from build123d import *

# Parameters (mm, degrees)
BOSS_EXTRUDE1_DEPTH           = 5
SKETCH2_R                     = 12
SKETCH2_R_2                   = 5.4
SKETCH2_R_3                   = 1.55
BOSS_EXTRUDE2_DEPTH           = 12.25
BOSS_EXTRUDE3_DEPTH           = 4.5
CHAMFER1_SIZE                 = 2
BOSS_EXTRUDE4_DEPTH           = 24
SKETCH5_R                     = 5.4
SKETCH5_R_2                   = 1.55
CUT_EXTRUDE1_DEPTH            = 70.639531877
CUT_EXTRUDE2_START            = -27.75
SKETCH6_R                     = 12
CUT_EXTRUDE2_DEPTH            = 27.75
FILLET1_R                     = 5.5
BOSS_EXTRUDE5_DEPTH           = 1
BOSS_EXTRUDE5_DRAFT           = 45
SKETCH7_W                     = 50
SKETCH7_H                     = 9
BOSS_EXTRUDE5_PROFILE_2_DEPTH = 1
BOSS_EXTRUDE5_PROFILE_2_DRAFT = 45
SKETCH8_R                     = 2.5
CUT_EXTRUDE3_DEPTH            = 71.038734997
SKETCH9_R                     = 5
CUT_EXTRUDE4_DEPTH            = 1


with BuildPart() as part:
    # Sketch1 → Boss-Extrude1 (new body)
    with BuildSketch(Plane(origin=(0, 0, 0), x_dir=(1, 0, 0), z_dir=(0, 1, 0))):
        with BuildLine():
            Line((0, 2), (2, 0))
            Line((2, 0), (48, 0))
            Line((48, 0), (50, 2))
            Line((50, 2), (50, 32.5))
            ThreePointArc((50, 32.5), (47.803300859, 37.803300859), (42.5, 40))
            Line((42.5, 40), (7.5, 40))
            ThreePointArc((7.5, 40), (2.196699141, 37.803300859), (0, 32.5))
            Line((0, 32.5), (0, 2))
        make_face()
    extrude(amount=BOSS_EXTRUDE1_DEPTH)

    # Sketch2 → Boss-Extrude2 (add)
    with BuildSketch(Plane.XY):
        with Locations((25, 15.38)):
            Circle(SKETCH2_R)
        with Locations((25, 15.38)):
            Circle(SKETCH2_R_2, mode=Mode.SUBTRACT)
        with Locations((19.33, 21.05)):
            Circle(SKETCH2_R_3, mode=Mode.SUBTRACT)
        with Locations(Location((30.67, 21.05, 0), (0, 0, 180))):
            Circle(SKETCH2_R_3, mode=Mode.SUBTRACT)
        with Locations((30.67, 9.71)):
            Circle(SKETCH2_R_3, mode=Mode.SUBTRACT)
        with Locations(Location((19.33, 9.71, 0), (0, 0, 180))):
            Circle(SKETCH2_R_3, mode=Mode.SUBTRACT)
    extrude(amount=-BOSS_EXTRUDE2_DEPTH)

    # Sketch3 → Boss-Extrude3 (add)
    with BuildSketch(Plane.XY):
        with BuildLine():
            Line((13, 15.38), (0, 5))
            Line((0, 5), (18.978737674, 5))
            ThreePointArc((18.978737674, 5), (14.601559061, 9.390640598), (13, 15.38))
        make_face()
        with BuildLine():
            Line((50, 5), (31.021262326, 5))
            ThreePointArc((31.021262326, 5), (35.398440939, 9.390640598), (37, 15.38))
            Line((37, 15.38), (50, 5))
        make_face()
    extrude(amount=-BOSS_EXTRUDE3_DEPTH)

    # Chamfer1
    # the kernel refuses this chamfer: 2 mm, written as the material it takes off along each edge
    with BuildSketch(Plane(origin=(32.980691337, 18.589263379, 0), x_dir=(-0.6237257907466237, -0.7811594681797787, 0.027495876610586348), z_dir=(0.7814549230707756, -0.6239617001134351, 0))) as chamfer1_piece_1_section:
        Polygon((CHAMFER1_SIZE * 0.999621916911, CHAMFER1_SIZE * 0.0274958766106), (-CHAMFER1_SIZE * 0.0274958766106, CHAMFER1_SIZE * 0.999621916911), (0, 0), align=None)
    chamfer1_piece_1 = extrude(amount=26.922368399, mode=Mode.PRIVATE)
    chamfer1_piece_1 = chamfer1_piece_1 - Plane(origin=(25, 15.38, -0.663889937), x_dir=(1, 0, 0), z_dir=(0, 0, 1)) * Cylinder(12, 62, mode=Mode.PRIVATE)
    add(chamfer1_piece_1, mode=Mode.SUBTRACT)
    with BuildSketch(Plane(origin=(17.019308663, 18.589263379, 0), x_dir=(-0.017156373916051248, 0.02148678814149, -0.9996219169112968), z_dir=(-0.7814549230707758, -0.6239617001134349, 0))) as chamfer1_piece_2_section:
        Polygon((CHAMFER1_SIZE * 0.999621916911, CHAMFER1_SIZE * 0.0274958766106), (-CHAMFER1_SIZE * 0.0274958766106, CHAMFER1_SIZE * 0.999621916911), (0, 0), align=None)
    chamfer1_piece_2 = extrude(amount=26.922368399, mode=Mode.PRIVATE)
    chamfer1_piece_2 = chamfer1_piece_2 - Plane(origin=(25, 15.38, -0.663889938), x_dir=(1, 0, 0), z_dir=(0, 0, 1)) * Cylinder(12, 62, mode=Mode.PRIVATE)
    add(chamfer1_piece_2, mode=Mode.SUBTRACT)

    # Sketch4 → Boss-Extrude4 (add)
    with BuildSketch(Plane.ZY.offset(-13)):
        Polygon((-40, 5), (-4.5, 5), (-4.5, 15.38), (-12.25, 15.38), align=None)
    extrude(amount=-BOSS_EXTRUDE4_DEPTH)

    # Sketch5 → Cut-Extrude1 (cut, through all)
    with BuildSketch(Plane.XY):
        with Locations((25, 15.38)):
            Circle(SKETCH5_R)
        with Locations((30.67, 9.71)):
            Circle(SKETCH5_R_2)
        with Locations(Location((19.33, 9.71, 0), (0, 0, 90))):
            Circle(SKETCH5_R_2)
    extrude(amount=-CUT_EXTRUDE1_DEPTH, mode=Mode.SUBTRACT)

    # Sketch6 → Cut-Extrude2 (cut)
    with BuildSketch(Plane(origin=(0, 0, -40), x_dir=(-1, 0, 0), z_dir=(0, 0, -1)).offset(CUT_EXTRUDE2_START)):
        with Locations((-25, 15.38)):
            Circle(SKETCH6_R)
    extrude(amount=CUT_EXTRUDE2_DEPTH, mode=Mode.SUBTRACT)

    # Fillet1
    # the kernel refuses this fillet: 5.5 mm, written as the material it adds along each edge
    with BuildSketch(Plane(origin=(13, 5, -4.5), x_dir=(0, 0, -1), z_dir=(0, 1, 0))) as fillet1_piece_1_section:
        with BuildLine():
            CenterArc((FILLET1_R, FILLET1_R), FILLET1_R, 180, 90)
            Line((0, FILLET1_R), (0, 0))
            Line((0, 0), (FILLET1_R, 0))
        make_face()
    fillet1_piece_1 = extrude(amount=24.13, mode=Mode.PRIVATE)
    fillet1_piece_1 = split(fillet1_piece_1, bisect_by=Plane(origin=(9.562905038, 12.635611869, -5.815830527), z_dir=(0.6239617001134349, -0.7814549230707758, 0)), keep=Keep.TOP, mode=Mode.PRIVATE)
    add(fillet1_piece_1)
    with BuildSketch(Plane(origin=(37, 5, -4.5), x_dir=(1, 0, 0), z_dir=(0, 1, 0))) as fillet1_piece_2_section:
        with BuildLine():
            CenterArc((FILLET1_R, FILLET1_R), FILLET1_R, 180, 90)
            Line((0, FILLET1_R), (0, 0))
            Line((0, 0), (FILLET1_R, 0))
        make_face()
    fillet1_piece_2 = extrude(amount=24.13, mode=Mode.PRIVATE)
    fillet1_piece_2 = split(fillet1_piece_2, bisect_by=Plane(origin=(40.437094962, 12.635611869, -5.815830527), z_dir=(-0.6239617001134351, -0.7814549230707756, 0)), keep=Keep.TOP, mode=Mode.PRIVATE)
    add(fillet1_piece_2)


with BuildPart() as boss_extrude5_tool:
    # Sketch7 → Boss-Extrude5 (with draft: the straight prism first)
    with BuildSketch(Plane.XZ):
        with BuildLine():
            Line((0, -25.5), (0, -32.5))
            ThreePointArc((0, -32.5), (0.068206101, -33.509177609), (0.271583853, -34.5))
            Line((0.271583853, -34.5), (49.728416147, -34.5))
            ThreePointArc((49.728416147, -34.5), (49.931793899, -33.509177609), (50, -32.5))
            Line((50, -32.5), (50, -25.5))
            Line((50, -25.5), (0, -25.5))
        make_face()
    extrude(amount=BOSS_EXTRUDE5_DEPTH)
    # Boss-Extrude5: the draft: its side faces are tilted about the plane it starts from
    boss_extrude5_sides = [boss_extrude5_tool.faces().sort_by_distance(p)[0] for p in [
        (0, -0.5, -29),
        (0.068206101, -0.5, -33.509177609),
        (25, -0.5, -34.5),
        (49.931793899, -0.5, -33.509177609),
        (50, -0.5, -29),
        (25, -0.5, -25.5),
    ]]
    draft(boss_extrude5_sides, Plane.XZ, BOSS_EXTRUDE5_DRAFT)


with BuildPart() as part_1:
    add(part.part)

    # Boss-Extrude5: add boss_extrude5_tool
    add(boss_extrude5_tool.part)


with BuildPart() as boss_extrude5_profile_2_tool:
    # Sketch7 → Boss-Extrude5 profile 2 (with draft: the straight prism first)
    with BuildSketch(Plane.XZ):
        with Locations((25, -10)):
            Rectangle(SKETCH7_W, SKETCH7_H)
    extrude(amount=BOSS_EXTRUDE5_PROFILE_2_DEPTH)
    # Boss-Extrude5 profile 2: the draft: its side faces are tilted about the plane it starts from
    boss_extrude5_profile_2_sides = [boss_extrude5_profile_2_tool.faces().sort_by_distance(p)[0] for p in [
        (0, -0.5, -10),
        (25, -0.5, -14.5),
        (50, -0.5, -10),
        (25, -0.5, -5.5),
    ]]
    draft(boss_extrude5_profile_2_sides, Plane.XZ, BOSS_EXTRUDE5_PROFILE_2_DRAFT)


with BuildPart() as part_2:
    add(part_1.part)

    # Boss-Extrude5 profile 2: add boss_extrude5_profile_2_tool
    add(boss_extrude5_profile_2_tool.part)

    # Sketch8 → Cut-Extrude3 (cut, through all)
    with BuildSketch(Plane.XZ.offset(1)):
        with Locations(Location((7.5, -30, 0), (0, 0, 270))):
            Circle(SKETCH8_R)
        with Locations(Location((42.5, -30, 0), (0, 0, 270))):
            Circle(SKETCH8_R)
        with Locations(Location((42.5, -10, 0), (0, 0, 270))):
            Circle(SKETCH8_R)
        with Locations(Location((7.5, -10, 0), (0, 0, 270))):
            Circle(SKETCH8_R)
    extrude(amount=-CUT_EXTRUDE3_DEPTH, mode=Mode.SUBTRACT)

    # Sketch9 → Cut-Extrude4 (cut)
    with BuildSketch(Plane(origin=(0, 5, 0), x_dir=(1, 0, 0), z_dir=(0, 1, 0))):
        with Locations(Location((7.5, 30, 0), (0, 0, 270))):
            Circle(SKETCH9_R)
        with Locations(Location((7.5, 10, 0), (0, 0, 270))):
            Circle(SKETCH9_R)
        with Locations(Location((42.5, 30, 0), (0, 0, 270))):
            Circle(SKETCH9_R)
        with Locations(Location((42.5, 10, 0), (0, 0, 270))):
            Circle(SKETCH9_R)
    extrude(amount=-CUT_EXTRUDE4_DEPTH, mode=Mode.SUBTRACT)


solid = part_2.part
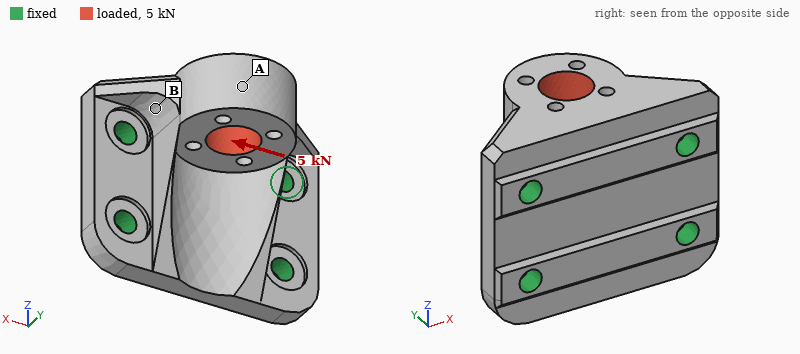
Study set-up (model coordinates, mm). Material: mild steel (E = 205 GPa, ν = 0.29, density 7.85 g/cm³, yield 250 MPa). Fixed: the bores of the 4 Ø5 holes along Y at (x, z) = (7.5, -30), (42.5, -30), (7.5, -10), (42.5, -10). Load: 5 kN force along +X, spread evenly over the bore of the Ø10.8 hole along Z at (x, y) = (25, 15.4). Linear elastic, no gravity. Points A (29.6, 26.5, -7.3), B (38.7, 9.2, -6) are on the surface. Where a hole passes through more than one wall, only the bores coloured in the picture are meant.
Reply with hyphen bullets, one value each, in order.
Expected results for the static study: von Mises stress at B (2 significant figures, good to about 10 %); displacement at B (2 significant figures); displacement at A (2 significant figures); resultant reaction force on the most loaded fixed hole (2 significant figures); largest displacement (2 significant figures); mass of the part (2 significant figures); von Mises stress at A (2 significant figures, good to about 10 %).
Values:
- 54 MPa
- 4.9 µm
- 12 µm
- 3.1 kN
- 12 µm
- 120 g
- 15 MPa
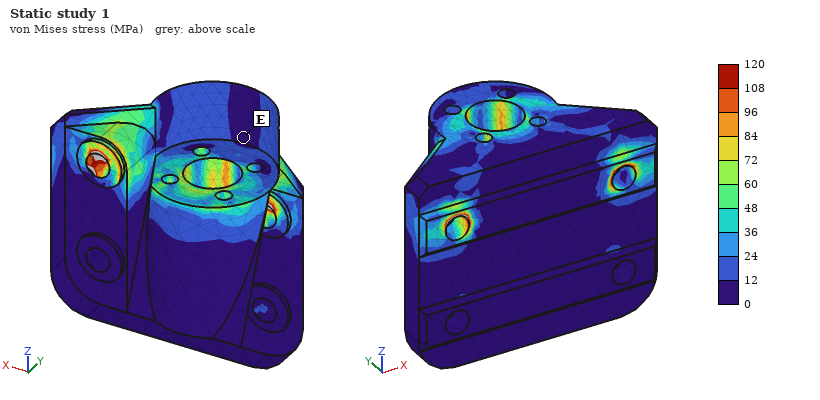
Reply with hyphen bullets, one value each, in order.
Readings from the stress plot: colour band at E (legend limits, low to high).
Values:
- 0 to 12 MPa
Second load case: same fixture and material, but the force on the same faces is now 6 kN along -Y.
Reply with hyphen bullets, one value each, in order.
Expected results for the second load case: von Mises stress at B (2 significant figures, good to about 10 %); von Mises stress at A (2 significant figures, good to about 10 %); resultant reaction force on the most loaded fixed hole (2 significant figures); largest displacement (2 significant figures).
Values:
- 54 MPa
- 17 MPa
- 3.5 kN
- 15 µm
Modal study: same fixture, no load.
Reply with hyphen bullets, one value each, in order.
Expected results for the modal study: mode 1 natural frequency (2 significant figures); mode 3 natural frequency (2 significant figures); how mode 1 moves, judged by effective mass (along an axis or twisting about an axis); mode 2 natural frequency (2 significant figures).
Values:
- 10 kHz
- 19 kHz
- along Z
- 19 kHz
